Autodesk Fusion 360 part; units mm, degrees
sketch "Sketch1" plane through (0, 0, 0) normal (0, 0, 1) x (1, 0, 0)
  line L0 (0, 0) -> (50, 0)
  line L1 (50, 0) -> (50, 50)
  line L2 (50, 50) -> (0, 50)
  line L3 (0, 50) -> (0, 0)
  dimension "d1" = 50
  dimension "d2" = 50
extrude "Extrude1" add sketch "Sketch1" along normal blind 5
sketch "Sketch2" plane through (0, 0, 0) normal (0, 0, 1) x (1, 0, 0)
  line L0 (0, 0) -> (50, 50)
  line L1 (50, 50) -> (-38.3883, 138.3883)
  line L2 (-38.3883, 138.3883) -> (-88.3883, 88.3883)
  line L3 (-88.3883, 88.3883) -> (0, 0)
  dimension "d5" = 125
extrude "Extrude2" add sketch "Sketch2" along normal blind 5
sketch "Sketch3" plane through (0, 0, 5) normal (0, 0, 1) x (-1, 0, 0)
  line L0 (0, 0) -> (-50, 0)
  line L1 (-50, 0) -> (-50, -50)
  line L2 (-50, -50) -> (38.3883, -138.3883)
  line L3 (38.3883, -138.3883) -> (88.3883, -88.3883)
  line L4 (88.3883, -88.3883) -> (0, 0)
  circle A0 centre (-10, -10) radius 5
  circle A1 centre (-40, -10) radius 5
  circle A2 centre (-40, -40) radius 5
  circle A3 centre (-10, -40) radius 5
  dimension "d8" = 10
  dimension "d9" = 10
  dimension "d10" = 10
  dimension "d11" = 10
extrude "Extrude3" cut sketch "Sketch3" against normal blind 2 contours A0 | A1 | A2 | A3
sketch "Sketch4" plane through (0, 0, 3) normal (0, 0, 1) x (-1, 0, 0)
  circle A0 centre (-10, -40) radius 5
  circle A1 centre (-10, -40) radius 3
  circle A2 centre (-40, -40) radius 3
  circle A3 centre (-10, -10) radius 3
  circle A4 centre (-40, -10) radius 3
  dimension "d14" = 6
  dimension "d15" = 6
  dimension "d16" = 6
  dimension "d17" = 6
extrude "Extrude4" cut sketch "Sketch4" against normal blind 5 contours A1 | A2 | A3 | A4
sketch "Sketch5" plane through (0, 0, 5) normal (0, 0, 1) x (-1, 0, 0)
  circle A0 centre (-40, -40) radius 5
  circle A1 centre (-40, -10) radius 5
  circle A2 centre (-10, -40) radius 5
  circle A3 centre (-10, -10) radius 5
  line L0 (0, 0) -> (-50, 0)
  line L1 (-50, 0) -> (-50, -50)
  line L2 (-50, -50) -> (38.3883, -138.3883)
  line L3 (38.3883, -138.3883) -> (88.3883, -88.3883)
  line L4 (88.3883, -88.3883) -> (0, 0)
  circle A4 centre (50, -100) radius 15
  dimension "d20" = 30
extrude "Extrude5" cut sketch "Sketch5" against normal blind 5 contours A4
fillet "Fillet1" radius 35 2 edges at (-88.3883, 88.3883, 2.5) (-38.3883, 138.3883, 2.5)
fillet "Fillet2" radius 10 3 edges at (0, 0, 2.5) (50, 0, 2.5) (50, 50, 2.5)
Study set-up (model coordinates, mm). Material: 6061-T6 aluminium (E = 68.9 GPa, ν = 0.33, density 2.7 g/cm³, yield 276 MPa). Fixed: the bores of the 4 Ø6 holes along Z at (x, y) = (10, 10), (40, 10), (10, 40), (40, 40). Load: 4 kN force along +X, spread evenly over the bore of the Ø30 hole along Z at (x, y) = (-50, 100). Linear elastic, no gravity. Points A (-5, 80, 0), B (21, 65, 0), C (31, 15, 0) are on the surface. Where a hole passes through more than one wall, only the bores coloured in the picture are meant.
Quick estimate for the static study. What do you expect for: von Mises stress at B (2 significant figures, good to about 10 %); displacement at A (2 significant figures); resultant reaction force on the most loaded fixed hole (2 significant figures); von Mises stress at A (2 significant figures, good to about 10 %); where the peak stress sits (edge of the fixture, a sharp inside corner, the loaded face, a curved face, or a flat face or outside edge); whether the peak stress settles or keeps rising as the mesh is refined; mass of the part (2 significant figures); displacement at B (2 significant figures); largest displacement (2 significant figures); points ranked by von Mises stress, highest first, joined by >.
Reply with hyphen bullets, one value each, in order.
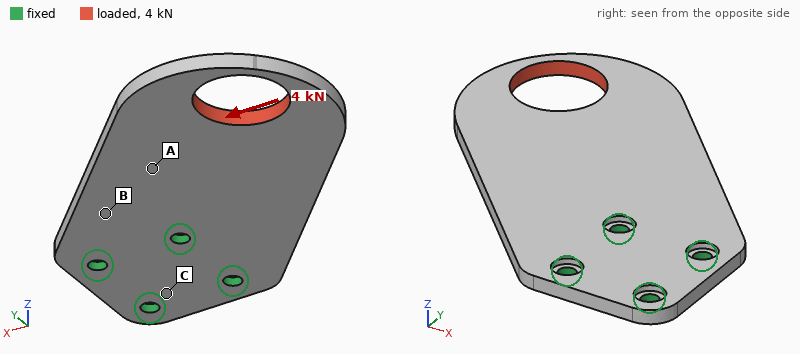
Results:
- 44 MPa
- 0.073 mm
- 4.7 kN
- 25 MPa
- edge of the fixture
- keeps rising
- 120 g
- 0.036 mm
- 0.23 mm
- B > A > C
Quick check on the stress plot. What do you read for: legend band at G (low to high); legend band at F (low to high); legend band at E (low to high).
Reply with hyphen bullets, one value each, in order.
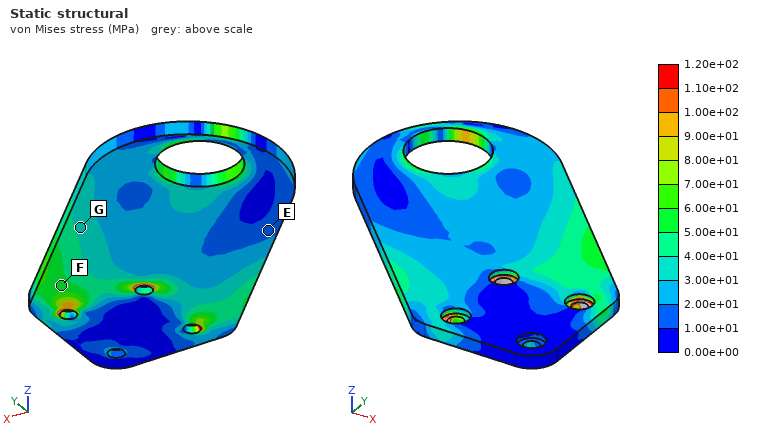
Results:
- 3.00e+01 to 4.00e+01 MPa
- 5.00e+01 to 6.00e+01 MPa
- 1.00e+01 to 2.00e+01 MPa
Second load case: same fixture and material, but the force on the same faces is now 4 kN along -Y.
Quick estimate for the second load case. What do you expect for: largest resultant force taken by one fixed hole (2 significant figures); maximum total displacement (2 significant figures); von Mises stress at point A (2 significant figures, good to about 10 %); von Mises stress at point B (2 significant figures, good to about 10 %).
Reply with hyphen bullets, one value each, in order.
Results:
- 4.7 kN
- 0.23 mm
- 17 MPa
- 32 MPa
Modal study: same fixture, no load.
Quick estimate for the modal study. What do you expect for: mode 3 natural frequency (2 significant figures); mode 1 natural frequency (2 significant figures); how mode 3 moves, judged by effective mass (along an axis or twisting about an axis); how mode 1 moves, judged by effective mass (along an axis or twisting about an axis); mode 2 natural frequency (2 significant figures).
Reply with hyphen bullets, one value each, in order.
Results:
- 2200 Hz
- 460 Hz
- along Z
- along Z
- 1100 Hz
